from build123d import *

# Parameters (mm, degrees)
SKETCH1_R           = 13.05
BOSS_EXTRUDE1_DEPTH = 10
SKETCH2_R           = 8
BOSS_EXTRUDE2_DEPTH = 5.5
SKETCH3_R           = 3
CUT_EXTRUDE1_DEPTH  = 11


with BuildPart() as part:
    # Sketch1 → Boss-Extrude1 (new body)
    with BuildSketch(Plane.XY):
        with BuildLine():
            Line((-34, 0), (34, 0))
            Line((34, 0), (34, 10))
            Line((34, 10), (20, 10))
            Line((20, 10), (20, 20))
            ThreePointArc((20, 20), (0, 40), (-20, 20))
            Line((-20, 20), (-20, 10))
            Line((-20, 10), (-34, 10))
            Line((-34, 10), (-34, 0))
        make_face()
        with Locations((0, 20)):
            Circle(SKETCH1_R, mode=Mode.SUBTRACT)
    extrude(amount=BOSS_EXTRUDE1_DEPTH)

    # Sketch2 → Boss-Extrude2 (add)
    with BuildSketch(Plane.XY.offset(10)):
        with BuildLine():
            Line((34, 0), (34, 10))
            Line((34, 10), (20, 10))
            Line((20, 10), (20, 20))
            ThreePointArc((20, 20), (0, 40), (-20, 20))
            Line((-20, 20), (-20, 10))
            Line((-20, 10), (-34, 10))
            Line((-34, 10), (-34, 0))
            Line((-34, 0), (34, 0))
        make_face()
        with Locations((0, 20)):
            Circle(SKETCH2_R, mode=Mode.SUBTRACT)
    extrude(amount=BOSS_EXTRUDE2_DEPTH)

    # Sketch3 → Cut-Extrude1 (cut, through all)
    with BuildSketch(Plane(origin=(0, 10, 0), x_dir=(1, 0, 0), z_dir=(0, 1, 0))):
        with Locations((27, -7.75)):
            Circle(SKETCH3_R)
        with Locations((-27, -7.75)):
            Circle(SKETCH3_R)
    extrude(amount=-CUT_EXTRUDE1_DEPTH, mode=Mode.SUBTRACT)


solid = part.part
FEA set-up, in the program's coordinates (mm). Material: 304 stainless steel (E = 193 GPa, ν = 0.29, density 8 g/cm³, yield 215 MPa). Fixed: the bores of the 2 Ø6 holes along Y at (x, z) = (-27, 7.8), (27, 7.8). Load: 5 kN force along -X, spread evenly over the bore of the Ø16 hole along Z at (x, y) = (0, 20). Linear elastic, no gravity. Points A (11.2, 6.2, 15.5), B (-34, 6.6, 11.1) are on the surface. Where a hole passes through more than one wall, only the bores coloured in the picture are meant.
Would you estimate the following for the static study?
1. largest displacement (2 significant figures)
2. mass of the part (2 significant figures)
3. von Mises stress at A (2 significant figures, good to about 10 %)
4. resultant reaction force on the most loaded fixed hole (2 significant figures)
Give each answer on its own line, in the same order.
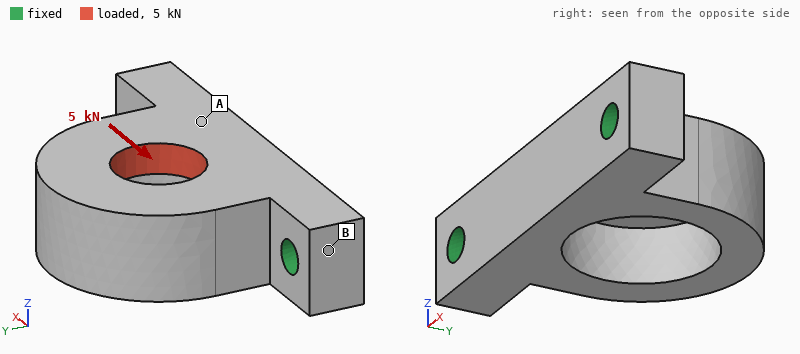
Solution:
11 µm
160 g
16 MPa
3.0 kN
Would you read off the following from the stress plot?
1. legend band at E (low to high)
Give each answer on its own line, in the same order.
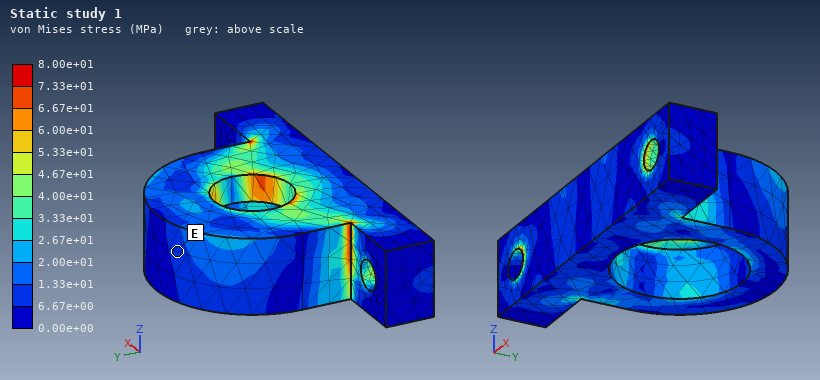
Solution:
6.67e+00 to 1.33e+01 MPa
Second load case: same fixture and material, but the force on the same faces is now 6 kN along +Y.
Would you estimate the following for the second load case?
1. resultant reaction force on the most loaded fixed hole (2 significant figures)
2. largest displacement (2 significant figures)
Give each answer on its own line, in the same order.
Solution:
3.1 kN
30 µm
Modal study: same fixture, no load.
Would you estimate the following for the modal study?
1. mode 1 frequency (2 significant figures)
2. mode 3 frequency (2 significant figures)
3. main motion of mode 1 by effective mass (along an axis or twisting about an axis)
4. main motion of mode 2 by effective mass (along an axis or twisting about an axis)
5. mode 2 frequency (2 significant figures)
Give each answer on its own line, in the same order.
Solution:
5000 Hz
15 kHz
along Z
along X
11 kHz
